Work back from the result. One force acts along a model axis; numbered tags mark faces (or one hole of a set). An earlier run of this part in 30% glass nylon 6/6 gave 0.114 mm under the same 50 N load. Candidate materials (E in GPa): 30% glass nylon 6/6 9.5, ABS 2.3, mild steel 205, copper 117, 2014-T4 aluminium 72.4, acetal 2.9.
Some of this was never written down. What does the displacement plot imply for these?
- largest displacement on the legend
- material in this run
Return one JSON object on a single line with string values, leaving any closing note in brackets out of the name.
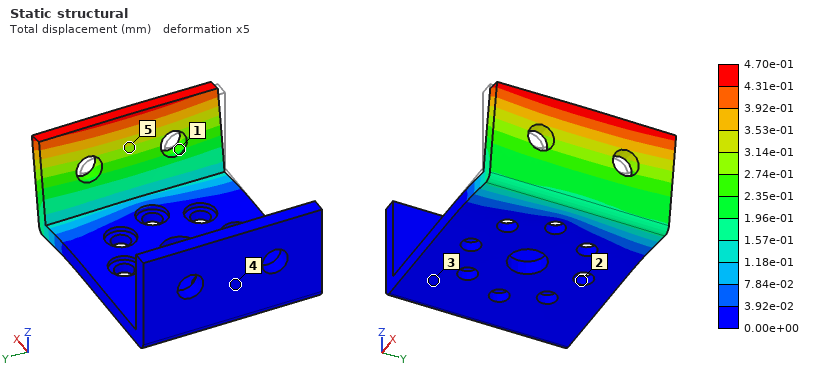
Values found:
{"largest displacement on the legend": "4.70e-01 mm", "material in this run": "ABS"}
